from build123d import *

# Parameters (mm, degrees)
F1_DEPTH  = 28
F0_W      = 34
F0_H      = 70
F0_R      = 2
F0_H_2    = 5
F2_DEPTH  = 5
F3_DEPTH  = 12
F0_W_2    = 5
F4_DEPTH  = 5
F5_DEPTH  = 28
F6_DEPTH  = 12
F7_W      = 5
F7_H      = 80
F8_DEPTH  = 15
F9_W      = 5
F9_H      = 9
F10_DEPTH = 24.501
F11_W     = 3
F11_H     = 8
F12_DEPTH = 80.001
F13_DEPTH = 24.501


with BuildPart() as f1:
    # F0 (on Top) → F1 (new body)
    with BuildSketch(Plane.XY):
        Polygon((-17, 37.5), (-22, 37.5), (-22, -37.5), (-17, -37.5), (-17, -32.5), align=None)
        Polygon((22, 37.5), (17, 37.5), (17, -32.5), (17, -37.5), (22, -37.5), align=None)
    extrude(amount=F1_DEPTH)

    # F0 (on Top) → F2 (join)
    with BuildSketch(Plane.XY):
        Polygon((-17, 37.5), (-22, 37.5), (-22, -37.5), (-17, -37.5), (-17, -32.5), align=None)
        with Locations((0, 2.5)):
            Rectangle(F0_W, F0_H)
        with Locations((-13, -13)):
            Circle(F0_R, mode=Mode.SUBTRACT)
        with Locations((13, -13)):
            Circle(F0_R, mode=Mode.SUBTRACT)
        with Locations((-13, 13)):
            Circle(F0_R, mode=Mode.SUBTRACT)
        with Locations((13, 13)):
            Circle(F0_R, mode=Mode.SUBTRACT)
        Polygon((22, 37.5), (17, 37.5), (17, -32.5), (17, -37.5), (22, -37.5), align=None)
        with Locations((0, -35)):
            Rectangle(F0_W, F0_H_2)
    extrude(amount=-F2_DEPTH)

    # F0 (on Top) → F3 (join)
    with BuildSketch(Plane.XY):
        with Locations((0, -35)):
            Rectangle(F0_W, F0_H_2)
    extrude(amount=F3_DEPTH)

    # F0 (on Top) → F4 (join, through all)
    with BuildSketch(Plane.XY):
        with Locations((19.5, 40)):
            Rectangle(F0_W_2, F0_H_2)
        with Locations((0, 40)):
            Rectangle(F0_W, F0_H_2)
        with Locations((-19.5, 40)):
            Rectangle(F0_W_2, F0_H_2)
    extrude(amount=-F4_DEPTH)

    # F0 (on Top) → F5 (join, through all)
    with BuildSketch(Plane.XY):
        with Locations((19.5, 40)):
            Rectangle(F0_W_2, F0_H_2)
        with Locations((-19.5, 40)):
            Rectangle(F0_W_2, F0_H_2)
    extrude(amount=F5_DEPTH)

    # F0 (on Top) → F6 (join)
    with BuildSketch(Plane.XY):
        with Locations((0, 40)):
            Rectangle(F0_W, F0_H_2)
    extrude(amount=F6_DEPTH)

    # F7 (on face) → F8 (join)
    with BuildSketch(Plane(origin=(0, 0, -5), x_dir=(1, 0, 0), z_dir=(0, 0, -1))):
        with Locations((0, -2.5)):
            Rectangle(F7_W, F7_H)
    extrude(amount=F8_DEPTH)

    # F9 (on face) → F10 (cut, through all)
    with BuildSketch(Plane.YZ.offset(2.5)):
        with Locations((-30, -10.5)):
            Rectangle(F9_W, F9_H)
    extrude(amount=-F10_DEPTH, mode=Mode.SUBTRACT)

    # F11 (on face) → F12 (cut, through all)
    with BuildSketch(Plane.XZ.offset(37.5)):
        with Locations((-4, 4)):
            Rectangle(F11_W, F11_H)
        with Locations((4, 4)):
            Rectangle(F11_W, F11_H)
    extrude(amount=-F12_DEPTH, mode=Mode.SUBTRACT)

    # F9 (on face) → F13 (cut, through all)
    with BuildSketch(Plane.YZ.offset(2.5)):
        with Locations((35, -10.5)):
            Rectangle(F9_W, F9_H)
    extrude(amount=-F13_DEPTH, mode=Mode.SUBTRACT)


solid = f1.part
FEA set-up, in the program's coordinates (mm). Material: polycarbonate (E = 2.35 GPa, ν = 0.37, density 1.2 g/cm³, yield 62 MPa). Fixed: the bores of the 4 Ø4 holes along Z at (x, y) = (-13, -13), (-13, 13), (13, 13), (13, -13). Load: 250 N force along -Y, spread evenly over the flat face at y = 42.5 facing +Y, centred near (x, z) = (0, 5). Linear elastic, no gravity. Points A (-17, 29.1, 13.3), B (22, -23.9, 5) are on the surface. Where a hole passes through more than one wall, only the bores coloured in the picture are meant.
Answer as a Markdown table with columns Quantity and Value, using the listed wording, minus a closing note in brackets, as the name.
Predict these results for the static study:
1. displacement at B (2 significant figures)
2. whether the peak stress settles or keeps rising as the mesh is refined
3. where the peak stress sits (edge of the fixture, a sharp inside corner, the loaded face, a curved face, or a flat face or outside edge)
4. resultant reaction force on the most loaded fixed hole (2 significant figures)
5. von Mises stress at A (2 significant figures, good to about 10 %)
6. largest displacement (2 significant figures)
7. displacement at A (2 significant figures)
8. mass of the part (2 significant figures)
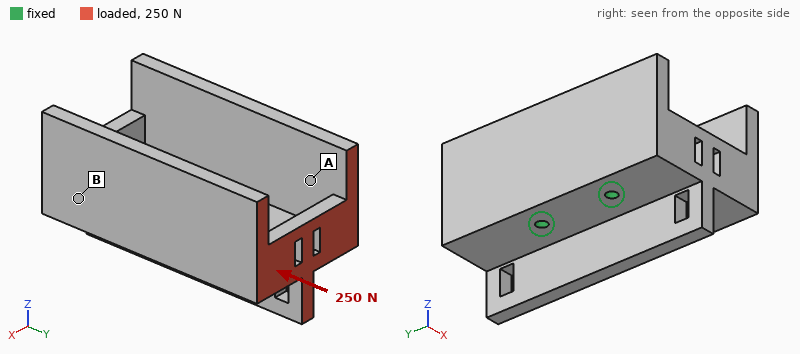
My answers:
| Quantity | Value |
|---|---|
| displacement at B | 13 µm |
| whether the peak stress settles or keeps rising as the mesh is refined | keeps rising |
| where the peak stress sits | edge of the fixture |
| resultant reaction force on the most loaded fixed hole | 91 N |
| von Mises stress at A | 0.79 MPa |
| largest displacement | 70 µm |
| displacement at A | 23 µm |
| mass of the part | 59 g |
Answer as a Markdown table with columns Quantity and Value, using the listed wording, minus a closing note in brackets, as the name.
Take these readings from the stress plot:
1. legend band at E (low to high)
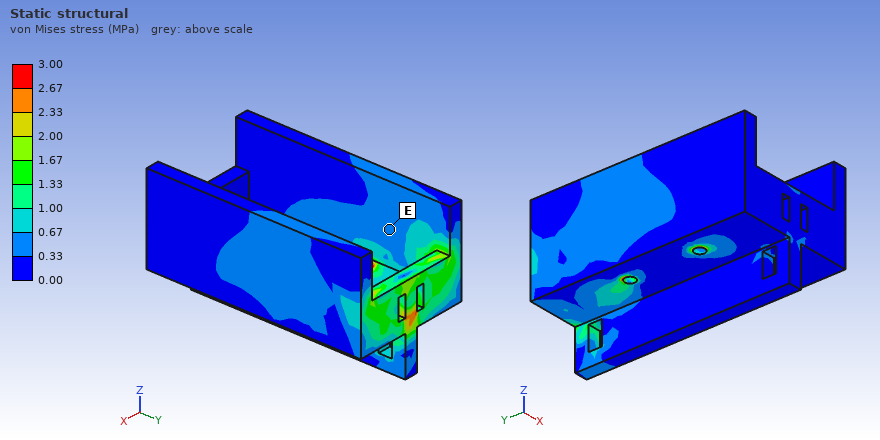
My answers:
| Quantity | Value |
|---|---|
| legend band at E | 0.33 to 0.67 MPa |
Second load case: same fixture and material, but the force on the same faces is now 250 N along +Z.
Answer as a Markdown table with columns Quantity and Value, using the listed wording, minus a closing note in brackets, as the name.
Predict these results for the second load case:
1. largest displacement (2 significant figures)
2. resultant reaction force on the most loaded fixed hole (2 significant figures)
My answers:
| Quantity | Value |
|---|---|
| largest displacement | 0.19 mm |
| resultant reaction force on the most loaded fixed hole | 250 N |
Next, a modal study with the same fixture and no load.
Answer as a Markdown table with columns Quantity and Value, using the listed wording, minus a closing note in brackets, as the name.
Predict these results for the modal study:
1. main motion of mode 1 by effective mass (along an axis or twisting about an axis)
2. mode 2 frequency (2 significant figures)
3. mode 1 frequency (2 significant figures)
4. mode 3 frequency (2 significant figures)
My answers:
| Quantity | Value |
|---|---|
| main motion of mode 1 by effective mass | along X |
| mode 2 frequency | 1300 Hz |
| mode 1 frequency | 1100 Hz |
| mode 3 frequency | 1300 Hz |
